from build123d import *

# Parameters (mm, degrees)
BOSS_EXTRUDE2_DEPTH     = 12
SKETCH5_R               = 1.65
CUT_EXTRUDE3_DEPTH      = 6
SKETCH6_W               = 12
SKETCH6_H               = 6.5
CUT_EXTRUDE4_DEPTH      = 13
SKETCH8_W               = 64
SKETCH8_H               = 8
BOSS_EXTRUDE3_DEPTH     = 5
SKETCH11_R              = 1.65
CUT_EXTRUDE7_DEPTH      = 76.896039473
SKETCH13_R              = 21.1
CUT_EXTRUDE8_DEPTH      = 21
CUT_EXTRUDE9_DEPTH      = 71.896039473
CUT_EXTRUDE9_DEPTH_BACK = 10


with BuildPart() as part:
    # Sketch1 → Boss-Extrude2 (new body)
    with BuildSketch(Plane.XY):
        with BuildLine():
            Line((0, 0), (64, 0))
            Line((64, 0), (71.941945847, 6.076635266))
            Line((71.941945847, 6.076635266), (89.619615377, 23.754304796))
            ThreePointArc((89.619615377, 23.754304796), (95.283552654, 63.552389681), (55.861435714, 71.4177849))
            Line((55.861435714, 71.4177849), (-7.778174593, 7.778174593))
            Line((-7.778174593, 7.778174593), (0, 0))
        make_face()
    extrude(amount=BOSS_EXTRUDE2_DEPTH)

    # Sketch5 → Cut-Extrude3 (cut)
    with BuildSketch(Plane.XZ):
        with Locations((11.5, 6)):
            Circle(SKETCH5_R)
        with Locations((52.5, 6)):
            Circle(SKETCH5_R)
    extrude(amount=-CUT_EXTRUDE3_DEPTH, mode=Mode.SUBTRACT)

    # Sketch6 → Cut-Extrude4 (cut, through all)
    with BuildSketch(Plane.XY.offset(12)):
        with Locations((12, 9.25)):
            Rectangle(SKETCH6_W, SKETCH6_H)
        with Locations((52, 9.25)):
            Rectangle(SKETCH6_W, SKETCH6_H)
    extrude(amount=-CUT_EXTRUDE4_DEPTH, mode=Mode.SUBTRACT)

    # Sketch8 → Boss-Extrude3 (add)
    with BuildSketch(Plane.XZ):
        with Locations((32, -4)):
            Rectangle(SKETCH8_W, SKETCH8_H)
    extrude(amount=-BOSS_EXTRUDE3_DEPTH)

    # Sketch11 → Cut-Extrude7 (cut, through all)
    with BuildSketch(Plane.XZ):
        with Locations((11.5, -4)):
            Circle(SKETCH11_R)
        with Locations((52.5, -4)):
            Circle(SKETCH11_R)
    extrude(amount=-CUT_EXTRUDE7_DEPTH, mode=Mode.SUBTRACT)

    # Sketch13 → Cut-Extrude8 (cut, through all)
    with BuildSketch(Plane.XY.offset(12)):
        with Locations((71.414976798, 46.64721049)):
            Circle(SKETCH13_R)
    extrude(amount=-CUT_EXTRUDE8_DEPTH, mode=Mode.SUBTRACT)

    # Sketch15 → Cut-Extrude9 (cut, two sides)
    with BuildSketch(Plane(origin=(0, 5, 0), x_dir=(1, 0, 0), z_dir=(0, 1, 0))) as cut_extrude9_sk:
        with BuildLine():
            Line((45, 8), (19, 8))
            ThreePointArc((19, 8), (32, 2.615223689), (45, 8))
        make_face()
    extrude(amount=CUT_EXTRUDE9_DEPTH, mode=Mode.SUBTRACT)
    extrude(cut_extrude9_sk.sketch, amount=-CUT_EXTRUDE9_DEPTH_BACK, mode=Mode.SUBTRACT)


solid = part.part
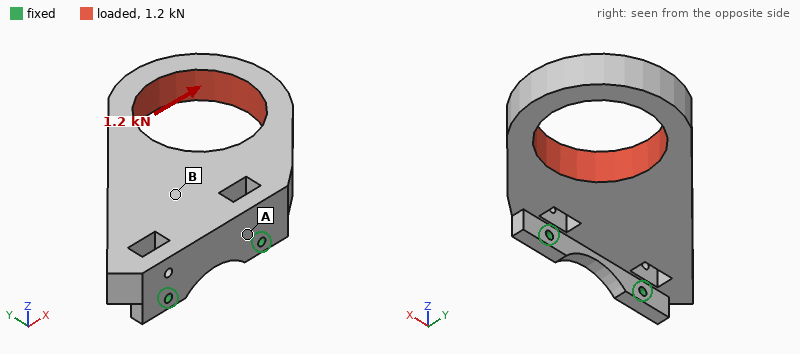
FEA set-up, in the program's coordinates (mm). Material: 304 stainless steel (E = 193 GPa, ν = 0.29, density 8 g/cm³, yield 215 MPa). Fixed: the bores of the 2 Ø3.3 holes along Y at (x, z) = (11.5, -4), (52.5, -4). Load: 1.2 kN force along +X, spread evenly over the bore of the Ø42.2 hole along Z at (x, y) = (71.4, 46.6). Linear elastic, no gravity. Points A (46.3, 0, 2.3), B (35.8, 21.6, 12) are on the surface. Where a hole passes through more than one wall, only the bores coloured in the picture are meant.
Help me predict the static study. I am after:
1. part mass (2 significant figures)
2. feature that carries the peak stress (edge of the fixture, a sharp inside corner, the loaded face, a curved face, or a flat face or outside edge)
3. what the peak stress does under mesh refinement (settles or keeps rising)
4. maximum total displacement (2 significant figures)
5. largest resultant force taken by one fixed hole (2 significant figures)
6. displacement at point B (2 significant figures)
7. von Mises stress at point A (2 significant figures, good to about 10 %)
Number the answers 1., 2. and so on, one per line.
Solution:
1. 350 g
2. edge of the fixture
3. keeps rising
4. 40 µm
5. 1.4 kN
6. 6.2 µm
7. 18 MPa
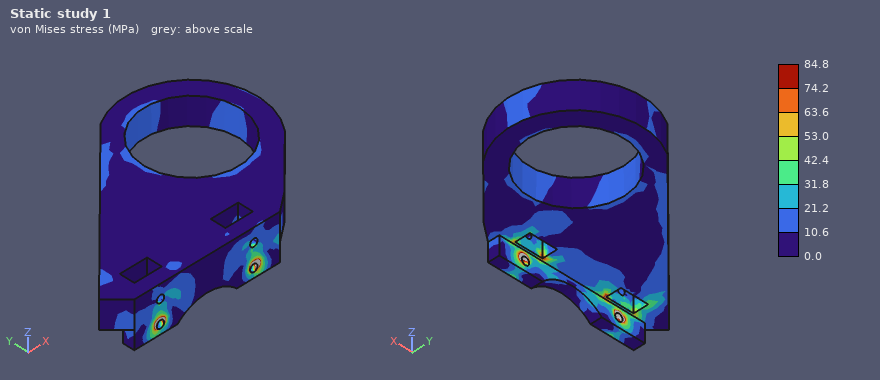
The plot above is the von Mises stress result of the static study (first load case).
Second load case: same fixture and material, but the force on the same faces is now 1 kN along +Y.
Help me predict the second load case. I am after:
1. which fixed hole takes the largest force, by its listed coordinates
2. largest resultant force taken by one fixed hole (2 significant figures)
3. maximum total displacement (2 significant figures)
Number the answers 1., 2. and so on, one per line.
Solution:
1. (52.5, -4)
2. 1.4 kN
3. 70 µm
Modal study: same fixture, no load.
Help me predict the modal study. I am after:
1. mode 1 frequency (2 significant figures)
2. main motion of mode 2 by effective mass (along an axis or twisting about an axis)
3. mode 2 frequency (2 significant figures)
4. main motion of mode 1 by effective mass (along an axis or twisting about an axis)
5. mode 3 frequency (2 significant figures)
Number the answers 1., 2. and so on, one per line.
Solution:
1. 740 Hz
2. along X
3. 2300 Hz
4. along Z
5. 2900 Hz
